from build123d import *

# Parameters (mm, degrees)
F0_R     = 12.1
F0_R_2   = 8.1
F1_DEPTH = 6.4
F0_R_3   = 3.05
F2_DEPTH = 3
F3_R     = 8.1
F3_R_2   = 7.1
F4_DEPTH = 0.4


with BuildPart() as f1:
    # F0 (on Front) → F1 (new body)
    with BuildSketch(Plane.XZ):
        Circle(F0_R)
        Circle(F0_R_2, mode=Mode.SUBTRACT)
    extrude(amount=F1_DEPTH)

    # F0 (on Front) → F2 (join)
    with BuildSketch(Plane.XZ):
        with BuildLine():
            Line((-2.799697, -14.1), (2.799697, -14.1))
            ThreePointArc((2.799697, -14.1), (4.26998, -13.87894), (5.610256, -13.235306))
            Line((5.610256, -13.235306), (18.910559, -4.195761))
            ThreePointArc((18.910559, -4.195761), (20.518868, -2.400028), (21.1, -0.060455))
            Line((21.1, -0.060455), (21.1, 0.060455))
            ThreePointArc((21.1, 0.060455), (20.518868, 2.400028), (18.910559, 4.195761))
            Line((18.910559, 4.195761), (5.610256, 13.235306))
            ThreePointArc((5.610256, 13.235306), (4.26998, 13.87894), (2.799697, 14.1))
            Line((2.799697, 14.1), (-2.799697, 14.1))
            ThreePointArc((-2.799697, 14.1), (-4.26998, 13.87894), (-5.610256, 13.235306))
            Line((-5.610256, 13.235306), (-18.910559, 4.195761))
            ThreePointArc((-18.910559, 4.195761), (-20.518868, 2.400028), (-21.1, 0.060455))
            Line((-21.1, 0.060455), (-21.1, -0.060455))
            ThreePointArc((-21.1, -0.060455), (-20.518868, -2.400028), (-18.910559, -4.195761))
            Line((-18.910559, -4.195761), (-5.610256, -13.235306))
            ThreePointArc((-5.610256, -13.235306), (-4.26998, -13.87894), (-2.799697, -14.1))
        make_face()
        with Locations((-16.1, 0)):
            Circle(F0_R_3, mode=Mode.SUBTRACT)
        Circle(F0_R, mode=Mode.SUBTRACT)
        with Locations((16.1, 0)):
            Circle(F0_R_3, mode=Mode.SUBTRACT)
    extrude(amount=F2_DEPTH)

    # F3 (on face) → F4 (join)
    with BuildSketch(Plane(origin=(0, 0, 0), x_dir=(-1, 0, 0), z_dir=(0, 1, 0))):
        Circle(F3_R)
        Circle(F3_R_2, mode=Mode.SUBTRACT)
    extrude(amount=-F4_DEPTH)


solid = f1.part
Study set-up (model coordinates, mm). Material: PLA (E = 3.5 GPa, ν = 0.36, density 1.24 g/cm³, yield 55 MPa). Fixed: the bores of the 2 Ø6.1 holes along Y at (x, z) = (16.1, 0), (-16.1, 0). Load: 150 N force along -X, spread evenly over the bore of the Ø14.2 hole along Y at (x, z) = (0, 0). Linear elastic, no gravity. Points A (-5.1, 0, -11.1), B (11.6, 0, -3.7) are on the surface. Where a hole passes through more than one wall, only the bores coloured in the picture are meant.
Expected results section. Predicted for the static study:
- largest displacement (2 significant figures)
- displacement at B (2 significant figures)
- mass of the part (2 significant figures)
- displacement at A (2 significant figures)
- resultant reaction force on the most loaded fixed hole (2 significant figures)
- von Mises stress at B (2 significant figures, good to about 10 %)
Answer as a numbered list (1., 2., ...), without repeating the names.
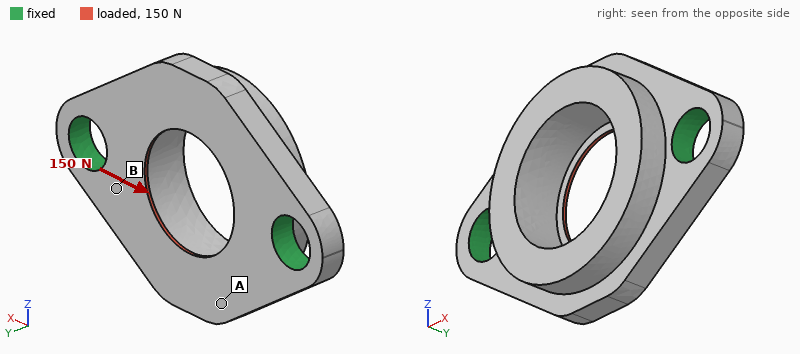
1. 17 µm
2. 2.9 µm
3. 3.1 g
4. 8.6 µm
5. 75 N
6. 2.5 MPa
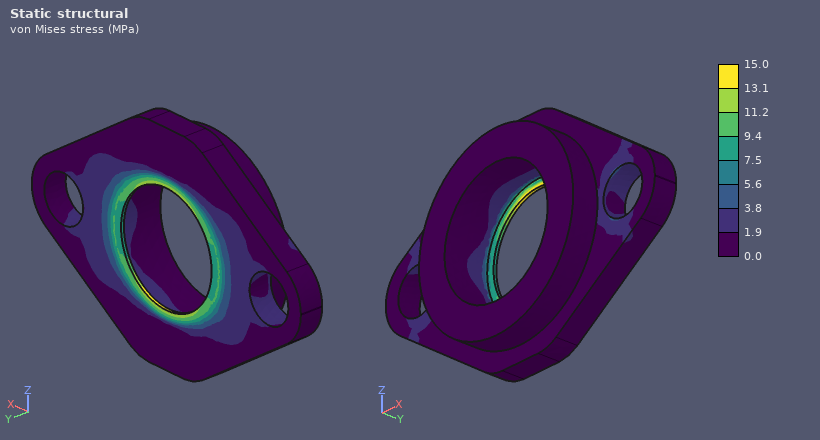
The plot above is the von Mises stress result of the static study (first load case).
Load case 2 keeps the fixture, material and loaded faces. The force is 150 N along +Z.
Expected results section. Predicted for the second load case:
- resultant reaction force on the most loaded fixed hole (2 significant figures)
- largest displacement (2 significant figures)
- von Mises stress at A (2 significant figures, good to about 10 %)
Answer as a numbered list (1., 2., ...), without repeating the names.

1. 75 N
2. 38 µm
3. 2.0 MPa
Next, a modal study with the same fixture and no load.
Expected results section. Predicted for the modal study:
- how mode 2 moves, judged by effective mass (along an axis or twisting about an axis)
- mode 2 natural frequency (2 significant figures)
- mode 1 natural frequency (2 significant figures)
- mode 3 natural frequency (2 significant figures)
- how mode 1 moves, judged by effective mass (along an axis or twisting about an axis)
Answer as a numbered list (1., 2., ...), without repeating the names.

1. along Y
2. 5200 Hz
3. 4000 Hz
4. 12 kHz
5. twisting about X
